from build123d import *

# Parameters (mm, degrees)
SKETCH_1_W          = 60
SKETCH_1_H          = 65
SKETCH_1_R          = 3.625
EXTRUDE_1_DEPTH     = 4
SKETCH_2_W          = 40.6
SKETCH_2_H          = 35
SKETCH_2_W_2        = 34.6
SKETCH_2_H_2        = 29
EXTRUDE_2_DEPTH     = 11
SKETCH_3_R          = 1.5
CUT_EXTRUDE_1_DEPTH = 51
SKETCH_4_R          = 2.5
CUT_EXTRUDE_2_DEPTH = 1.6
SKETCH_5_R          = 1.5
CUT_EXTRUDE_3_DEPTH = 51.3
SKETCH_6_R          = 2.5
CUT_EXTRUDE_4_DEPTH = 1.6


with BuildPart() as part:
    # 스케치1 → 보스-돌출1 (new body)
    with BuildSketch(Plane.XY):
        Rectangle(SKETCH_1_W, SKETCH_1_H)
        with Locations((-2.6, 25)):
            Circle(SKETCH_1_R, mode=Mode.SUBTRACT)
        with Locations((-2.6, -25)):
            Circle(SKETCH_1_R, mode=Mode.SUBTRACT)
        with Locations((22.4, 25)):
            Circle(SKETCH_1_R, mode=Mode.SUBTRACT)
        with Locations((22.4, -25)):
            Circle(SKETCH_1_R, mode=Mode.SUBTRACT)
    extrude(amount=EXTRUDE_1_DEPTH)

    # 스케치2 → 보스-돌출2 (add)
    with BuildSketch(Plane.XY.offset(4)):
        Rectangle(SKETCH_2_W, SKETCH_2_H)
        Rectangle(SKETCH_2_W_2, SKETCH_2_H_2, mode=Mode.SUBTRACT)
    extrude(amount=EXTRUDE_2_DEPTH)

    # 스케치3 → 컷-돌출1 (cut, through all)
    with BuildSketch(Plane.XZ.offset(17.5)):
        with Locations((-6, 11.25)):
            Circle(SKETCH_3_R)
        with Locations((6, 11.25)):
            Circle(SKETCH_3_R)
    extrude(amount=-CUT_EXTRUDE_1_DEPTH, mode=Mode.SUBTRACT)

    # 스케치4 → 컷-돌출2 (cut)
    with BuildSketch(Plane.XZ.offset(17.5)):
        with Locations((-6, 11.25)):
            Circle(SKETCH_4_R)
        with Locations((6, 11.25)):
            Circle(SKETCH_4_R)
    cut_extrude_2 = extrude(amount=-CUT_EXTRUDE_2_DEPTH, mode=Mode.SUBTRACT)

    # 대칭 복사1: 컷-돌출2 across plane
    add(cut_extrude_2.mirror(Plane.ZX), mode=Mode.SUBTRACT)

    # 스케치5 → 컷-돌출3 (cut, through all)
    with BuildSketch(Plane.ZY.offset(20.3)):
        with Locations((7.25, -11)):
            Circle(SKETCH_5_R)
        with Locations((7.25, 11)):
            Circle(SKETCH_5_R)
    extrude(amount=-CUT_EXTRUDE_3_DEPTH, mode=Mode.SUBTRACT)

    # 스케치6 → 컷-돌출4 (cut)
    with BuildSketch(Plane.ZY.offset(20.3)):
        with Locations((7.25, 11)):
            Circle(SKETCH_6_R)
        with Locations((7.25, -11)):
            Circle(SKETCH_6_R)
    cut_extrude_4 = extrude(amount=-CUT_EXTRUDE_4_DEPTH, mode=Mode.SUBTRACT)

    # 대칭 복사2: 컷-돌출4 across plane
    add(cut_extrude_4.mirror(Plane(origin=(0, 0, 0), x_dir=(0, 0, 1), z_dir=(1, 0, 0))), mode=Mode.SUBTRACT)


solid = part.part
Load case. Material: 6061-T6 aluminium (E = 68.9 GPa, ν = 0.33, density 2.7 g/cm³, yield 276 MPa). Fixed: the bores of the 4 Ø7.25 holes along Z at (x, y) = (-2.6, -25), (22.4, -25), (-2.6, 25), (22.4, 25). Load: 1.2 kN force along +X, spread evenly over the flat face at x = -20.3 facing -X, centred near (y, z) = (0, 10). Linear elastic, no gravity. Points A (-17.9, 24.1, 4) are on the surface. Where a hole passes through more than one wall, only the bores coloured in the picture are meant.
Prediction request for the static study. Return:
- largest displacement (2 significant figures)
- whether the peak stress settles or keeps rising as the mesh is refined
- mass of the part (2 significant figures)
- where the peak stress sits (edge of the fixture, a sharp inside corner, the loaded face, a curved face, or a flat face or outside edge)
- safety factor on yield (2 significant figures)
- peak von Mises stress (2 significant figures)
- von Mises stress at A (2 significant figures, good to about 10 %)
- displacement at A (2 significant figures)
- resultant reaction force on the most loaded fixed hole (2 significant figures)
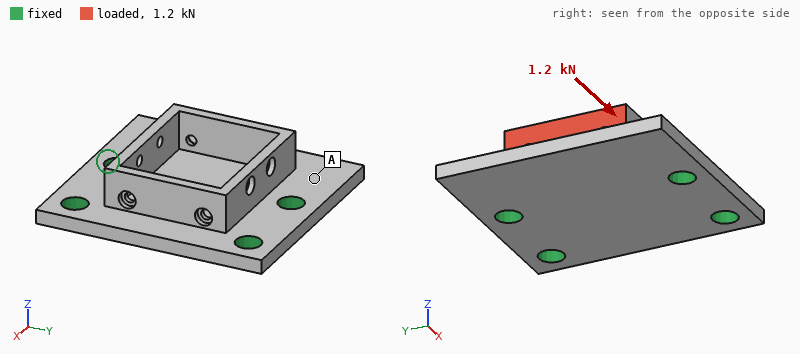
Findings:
61 µm
settles
52 g
a curved face
3.3
83 MPa
6.8 MPa
9.8 µm
390 N
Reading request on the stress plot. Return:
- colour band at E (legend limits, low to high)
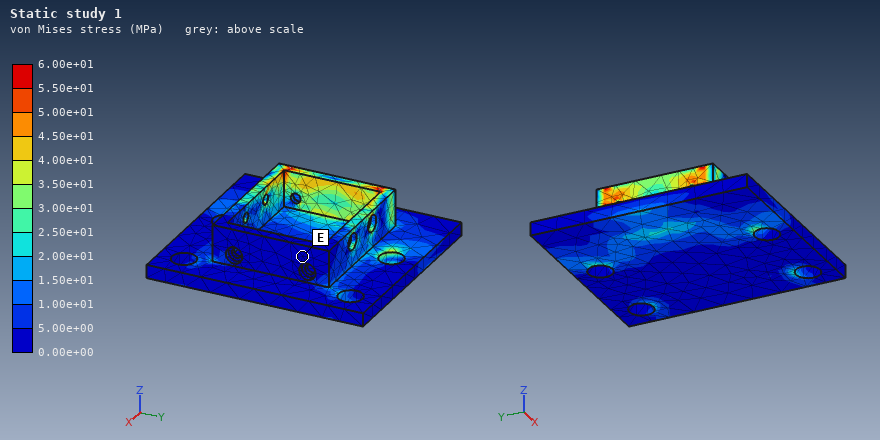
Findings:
0.00e+00 to 5.00e+00 MPa
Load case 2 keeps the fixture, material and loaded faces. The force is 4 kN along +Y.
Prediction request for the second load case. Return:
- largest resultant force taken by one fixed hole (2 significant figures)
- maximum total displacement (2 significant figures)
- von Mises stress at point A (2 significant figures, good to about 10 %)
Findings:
2.4 kN
59 µm
28 MPa
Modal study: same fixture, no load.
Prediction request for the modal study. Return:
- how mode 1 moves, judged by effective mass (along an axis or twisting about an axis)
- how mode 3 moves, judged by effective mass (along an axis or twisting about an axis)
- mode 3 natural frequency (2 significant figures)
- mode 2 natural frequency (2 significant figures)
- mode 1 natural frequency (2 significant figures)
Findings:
along Z
along Z
11 kHz
8100 Hz
5800 Hz
